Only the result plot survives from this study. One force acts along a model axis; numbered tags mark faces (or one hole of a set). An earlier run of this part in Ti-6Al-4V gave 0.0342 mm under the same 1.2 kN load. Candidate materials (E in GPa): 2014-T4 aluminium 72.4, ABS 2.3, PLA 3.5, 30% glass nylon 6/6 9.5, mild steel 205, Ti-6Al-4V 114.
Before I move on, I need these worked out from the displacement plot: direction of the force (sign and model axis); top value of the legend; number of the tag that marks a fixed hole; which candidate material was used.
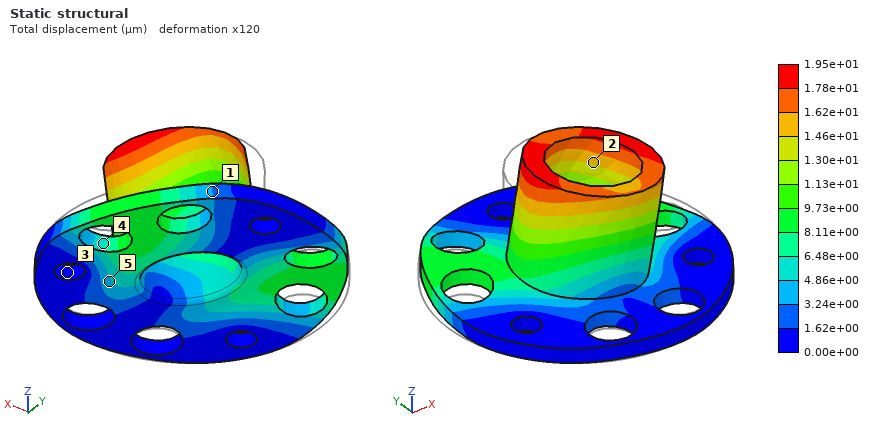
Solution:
+X
1.95e+01 µm
3
mild steel
